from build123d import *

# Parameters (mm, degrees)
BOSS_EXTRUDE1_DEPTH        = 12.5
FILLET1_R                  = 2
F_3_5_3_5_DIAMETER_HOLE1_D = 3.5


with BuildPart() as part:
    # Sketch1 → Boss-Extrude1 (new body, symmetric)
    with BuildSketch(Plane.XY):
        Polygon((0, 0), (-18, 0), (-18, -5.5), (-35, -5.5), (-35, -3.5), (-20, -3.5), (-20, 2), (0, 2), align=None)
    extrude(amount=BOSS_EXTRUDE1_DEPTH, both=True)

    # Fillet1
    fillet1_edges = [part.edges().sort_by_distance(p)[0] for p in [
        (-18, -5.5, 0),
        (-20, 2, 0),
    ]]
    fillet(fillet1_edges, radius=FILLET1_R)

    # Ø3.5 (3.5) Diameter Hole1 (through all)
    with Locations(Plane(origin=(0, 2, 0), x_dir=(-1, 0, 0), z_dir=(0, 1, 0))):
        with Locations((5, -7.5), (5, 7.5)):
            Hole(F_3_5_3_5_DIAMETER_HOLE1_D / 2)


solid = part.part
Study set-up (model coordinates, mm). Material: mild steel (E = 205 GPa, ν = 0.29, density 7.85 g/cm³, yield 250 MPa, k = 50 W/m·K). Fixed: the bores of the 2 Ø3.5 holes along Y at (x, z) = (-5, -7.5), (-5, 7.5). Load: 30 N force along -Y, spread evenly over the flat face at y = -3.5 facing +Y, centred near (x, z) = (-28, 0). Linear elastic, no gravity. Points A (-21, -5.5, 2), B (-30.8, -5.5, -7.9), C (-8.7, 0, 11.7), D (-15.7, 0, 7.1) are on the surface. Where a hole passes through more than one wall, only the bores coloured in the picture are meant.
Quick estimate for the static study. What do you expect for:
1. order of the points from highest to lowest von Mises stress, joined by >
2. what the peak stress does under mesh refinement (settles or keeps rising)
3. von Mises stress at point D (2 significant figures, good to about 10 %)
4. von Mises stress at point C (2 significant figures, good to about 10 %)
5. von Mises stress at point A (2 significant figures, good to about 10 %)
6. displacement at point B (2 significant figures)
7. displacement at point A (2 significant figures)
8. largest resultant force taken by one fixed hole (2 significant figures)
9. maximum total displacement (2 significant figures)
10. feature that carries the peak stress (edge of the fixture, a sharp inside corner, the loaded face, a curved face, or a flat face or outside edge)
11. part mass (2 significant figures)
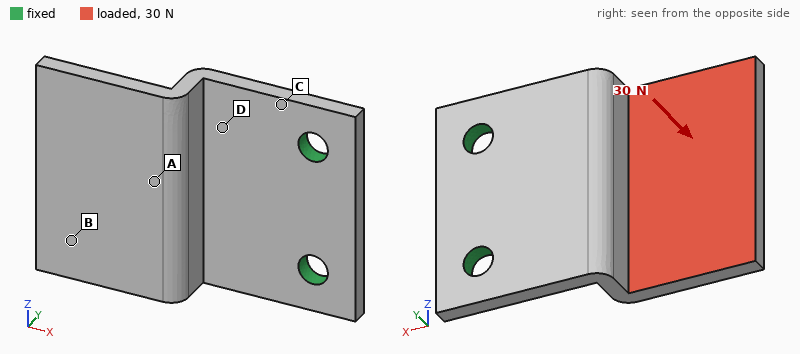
C > D > A > B
keeps rising
19 MPa
32 MPa
11 MPa
42 µm
21 µm
15 N
51 µm
edge of the fixture
15 g
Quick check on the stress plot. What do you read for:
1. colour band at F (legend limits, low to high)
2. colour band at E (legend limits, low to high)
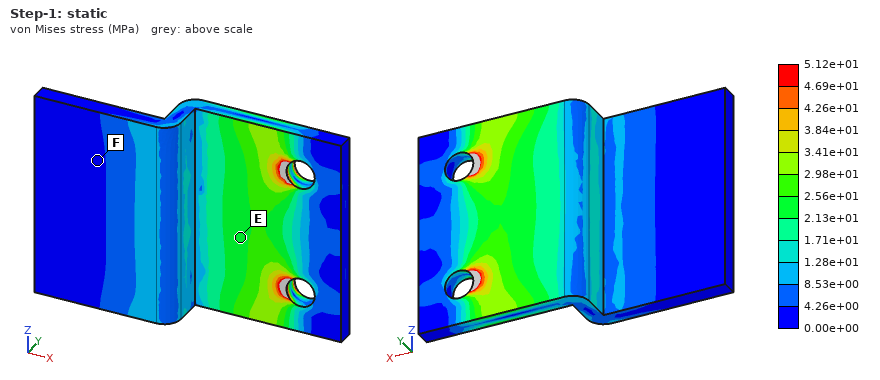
0.00e+00 to 4.26e+00 MPa
2.13e+01 to 2.56e+01 MPa
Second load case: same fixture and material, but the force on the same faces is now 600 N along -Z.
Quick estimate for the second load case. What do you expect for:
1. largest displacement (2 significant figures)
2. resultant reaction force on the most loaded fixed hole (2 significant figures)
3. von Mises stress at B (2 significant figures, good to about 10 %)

44 µm
840 N
18 MPa
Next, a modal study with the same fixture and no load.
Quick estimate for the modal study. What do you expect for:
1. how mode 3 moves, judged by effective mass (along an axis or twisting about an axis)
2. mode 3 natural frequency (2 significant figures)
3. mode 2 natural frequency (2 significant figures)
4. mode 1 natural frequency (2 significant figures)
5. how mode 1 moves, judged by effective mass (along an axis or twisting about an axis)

along Z
8200 Hz
5100 Hz
1700 Hz
along Y
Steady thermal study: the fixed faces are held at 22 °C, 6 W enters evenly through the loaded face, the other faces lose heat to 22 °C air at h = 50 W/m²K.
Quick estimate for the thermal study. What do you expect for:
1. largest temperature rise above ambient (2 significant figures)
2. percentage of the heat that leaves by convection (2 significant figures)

47 K
32 %
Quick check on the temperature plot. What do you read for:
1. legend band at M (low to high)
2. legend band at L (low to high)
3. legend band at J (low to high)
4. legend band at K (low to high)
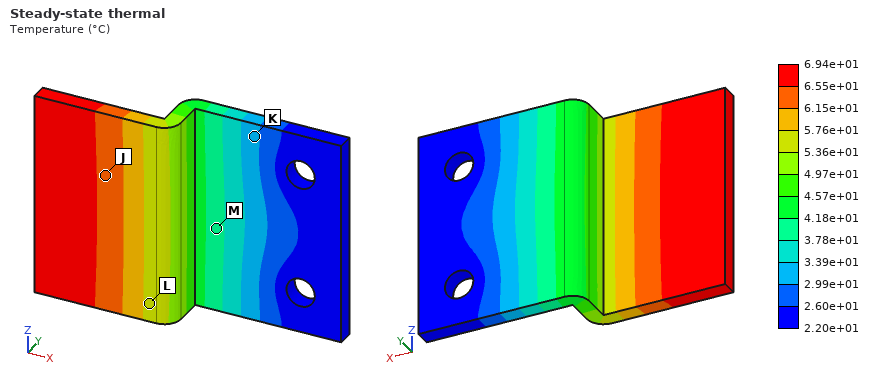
3.78e+01 to 4.18e+01 °C
5.36e+01 to 5.76e+01 °C
6.15e+01 to 6.55e+01 °C
2.99e+01 to 3.39e+01 °C
